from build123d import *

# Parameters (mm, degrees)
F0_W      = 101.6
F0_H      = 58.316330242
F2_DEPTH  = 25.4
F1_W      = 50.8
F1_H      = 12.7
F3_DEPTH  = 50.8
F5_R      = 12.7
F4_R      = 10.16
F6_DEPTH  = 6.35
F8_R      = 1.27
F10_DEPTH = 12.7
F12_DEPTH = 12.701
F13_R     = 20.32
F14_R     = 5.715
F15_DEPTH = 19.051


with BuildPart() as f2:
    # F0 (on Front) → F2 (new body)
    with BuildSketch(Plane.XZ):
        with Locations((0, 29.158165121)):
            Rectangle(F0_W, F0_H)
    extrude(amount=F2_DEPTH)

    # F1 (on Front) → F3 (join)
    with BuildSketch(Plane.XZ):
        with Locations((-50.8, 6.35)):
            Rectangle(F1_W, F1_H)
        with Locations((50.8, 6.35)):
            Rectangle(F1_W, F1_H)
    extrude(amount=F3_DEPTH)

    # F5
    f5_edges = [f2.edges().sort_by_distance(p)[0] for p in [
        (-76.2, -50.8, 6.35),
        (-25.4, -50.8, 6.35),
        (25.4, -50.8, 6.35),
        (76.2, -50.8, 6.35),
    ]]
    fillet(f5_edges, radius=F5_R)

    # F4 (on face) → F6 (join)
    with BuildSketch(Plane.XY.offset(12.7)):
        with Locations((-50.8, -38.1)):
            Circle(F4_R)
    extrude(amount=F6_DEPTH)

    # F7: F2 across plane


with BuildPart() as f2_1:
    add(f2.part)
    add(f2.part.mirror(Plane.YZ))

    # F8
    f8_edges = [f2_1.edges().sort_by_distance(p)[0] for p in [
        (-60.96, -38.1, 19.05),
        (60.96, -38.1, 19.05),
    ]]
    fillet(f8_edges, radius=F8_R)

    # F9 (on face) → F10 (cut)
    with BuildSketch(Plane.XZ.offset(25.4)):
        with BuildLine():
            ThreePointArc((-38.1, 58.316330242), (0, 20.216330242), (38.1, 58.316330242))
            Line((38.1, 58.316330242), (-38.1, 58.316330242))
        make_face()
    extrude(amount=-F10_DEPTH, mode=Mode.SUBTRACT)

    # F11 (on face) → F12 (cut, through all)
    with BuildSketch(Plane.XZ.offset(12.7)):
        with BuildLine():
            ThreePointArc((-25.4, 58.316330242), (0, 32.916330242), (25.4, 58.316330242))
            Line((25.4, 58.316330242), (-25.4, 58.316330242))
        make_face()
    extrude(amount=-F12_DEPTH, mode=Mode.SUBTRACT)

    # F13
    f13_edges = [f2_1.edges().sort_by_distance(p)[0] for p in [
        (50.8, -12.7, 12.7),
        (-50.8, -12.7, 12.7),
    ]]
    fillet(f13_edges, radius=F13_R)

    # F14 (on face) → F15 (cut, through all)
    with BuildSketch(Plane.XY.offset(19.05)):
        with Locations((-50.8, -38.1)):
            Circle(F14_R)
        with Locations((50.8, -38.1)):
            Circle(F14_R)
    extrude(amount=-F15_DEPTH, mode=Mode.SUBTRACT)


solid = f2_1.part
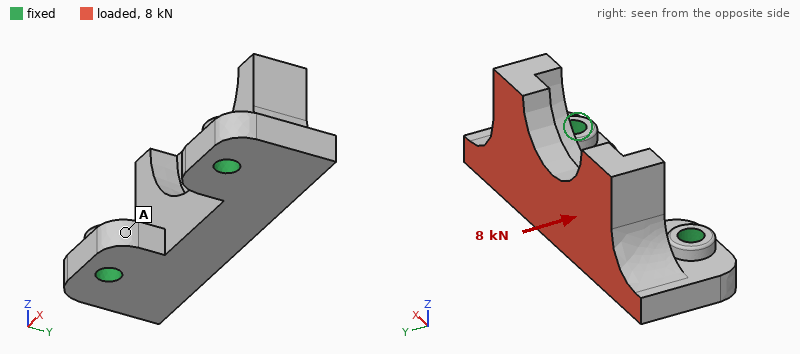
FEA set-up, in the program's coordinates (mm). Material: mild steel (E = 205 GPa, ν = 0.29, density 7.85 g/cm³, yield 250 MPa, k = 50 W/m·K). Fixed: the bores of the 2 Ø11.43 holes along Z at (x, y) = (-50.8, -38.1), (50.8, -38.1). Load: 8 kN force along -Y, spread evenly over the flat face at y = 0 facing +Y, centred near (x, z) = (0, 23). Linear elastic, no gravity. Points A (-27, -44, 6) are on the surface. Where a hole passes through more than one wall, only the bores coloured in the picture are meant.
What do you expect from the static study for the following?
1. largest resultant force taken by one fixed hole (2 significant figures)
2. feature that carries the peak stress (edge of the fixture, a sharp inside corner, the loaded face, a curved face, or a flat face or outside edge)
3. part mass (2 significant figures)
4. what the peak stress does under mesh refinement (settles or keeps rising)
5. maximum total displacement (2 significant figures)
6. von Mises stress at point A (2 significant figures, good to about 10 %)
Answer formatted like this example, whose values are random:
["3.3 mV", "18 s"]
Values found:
["4.3 kN", "a sharp inside corner", "1.3 kg", "keeps rising", "47 µm", "9.0 MPa"]
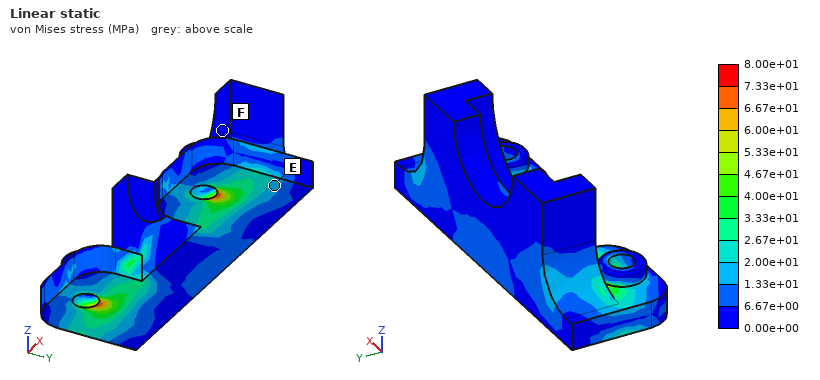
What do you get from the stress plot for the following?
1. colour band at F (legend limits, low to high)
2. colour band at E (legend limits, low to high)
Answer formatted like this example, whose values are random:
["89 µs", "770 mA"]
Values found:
["0.00e+00 to 6.67e+00 MPa", "1.33e+01 to 2.00e+01 MPa"]
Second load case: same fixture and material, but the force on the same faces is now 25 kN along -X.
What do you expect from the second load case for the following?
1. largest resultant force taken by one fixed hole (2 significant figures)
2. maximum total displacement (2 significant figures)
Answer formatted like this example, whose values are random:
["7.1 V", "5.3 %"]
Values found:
["15 kN", "25 µm"]
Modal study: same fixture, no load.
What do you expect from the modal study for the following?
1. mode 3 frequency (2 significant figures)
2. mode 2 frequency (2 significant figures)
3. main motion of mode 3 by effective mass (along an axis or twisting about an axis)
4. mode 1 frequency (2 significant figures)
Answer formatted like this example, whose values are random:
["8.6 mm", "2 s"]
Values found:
["6500 Hz", "4400 Hz", "along Z", "2400 Hz"]
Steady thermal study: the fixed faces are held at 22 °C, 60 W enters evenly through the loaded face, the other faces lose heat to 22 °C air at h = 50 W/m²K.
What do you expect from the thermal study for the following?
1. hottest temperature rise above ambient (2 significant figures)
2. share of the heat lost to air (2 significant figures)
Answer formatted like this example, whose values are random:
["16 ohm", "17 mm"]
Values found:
["26 K", "28 %"]
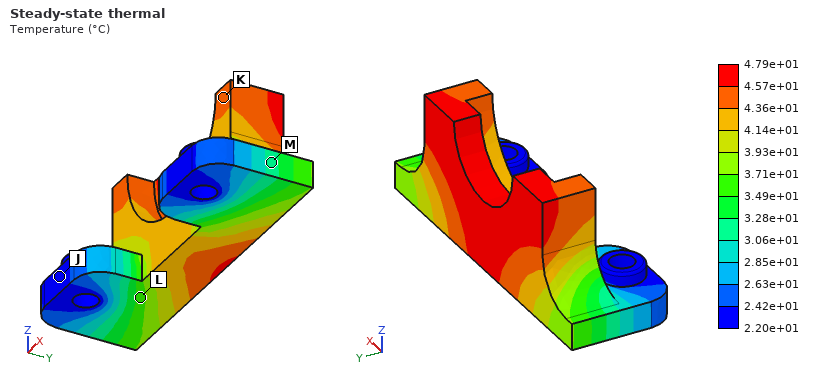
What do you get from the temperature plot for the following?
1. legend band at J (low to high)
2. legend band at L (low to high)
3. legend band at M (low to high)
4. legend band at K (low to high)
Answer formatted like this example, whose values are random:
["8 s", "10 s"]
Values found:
["2.20e+01 to 2.42e+01 °C", "3.49e+01 to 3.71e+01 °C", "3.06e+01 to 3.28e+01 °C", "4.36e+01 to 4.57e+01 °C"]
